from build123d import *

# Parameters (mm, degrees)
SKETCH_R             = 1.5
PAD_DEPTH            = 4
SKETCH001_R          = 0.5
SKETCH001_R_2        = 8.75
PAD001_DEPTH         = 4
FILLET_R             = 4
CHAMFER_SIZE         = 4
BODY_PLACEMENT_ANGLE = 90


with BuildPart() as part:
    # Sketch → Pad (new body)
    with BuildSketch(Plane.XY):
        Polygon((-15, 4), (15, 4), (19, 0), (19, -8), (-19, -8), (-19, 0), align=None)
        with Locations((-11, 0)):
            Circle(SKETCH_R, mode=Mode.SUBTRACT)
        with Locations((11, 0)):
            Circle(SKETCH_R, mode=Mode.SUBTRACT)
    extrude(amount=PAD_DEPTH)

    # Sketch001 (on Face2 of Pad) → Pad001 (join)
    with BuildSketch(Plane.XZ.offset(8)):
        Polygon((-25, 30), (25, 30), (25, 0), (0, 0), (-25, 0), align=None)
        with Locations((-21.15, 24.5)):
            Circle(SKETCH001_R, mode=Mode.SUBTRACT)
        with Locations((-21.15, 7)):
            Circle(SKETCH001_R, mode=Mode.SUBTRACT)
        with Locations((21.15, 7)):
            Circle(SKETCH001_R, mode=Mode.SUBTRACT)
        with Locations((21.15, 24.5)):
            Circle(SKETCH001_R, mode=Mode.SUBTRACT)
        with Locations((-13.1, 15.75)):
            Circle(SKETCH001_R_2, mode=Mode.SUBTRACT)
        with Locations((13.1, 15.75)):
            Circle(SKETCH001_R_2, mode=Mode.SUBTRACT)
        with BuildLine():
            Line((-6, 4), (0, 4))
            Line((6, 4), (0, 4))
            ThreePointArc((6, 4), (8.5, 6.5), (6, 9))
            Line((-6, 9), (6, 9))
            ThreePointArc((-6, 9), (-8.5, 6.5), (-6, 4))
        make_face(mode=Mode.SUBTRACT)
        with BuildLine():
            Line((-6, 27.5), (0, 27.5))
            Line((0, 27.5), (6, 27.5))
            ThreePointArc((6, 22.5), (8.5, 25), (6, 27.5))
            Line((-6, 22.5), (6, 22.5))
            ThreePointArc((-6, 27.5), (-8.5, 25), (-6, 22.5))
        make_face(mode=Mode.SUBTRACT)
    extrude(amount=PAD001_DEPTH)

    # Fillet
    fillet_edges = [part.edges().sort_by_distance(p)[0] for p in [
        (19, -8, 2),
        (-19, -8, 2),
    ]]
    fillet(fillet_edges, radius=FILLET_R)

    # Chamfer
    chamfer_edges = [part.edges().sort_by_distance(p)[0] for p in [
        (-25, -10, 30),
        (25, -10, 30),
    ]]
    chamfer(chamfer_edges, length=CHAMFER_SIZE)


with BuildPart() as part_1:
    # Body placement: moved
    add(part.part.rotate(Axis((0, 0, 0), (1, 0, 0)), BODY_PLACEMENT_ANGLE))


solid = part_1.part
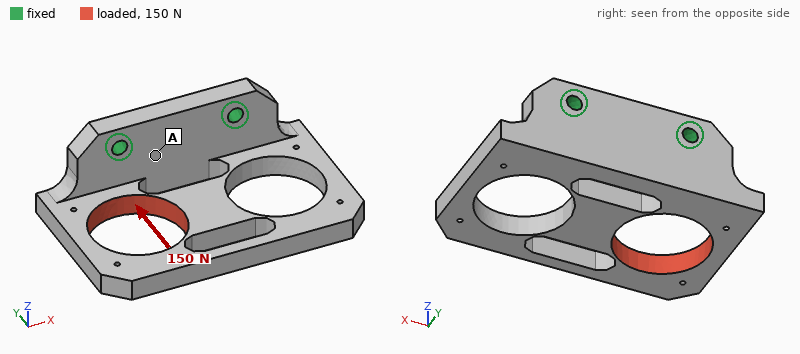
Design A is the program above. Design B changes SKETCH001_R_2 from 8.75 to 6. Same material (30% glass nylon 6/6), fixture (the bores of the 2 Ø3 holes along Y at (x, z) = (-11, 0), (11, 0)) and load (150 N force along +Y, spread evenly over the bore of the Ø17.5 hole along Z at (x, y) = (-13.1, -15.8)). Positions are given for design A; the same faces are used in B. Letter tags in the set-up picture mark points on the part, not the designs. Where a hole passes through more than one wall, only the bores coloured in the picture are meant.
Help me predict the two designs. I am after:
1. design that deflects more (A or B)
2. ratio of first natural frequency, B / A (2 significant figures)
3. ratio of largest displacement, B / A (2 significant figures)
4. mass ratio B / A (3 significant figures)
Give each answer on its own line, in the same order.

A
1.1
0.87
1.20
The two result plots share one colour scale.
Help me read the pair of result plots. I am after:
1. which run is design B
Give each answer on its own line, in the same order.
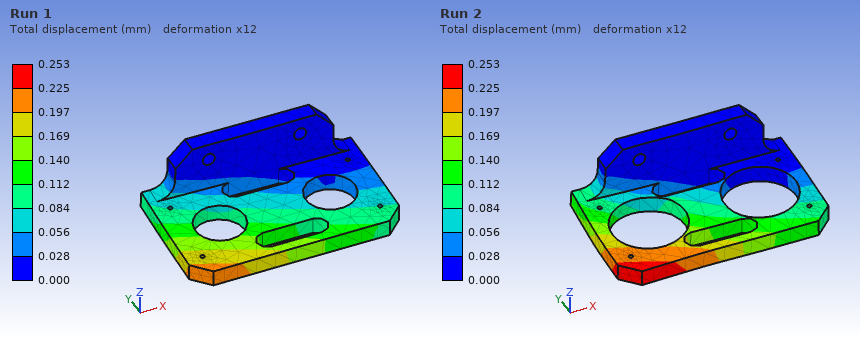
Run 1
